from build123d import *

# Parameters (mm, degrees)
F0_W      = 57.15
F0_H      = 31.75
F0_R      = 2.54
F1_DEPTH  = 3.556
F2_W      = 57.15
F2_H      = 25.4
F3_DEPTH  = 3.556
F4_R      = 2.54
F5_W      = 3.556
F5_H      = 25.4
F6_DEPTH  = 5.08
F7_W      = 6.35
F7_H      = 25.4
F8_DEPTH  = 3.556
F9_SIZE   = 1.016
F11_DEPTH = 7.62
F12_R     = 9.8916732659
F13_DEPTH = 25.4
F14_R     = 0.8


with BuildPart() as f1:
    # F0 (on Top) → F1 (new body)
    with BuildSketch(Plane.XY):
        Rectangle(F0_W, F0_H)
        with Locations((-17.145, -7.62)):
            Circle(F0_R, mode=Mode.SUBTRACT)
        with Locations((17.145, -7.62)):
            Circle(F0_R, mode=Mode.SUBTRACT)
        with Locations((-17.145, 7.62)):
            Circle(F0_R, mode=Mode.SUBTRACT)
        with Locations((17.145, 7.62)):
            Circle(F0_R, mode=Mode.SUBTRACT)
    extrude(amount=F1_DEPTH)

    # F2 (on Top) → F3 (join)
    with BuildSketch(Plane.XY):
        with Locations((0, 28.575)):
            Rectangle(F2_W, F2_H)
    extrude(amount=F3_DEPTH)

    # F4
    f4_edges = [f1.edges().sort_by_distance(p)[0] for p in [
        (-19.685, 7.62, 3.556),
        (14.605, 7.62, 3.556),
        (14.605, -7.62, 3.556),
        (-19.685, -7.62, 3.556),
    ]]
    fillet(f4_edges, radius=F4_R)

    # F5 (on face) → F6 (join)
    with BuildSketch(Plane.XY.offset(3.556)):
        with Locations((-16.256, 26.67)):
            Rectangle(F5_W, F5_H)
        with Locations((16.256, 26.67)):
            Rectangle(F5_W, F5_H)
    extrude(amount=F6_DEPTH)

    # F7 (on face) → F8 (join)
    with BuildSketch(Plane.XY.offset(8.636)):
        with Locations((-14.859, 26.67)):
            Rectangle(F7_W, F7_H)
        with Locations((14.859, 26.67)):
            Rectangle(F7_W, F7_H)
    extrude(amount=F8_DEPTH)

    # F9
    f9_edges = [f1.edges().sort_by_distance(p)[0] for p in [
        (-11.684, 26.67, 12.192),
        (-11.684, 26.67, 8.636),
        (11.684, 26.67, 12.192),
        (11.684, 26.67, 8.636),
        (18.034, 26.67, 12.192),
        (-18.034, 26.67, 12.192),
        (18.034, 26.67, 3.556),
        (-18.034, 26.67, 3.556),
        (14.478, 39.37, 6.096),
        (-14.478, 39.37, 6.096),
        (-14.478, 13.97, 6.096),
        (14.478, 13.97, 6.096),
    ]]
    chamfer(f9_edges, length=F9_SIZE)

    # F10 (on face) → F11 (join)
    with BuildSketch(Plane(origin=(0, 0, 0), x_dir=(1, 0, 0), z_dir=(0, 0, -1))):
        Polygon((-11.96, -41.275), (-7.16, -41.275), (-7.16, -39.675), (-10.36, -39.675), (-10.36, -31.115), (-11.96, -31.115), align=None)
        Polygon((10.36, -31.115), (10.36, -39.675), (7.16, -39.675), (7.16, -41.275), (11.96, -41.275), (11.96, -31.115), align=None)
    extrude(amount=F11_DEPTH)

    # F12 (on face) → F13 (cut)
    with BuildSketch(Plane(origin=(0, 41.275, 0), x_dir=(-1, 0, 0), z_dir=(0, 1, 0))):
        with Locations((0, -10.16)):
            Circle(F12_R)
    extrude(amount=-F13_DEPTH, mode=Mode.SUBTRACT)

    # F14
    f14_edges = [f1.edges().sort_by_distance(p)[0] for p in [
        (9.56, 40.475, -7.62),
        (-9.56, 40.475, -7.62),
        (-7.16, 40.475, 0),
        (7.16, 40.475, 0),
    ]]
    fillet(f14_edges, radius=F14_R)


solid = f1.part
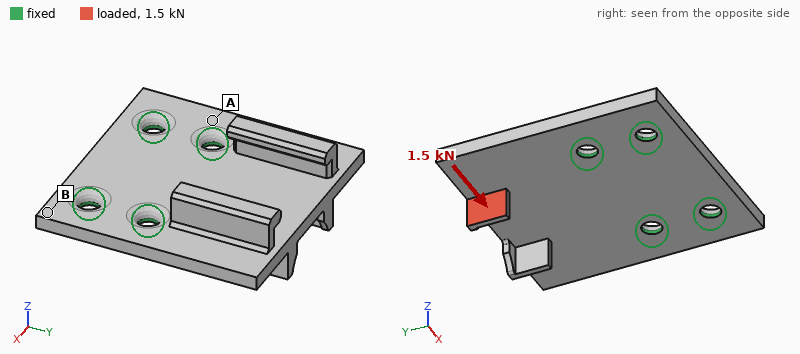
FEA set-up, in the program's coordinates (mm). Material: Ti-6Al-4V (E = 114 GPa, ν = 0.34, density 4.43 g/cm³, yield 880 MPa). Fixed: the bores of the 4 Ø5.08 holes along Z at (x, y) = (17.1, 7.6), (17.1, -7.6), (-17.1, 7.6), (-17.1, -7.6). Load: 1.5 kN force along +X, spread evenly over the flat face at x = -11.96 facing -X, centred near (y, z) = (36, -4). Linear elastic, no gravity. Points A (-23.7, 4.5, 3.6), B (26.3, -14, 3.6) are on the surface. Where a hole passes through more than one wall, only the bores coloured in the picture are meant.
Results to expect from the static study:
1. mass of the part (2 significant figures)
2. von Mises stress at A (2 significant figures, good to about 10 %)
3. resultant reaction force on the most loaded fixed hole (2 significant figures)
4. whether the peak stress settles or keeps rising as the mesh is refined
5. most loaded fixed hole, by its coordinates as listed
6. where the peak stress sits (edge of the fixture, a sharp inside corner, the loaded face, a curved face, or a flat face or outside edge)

60 g
71 MPa
1.3 kN
keeps rising
(-17.1, 7.6)
a sharp inside corner
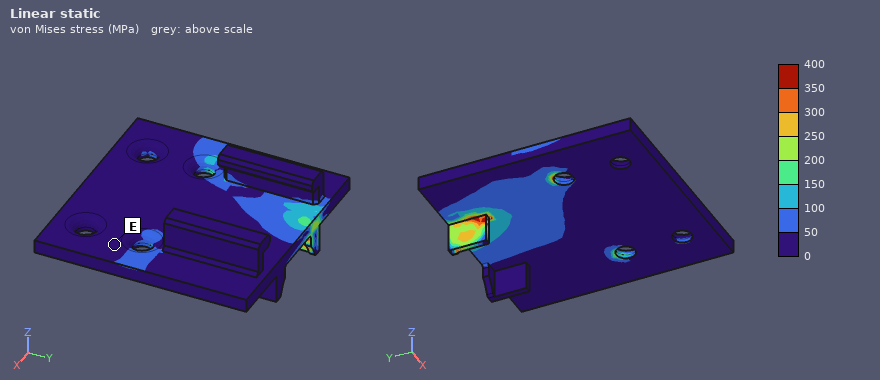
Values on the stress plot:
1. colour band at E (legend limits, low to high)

0 to 50 MPa
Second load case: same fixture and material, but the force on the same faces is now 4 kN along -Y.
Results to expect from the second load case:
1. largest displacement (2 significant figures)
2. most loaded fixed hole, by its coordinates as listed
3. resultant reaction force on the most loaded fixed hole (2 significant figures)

0.60 mm
(-17.1, 7.6)
3.4 kN
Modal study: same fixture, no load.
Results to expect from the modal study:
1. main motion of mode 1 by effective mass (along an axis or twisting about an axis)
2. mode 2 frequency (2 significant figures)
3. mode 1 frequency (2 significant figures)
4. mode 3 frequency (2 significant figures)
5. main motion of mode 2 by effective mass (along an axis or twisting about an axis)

along Z
3400 Hz
1900 Hz
7000 Hz
twisting about Y
